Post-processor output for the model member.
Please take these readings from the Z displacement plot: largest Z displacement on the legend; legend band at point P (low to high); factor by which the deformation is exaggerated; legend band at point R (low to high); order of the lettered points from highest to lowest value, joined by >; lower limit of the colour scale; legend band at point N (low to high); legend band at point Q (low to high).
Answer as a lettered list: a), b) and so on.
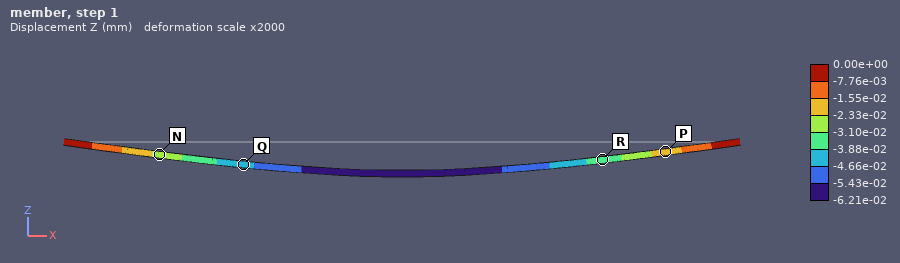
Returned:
a) 0.00e+00 mm
b) -2.33e-02 to -1.55e-02 mm
c) 2000
d) -3.88e-02 to -3.10e-02 mm
e) P > N > R > Q
f) -6.21e-02 mm
g) -3.10e-02 to -2.33e-02 mm
h) -4.66e-02 to -3.88e-02 mm
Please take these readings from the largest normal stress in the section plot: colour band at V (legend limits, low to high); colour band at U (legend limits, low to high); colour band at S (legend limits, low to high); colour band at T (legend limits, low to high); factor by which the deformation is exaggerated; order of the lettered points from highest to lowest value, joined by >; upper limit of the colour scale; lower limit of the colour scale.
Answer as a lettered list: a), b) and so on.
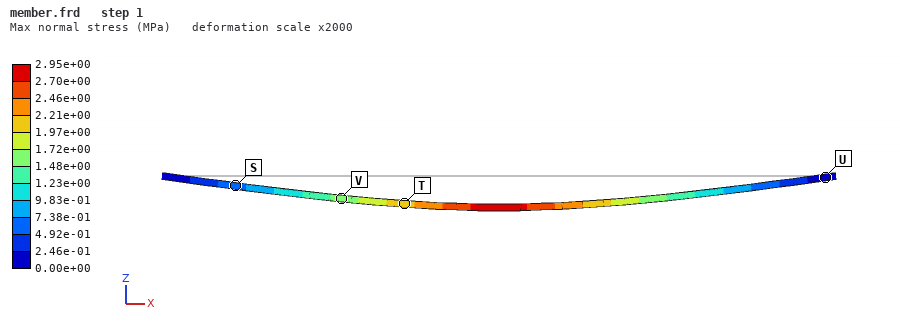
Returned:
a) 1.48e+00 to 1.72e+00 MPa
b) 0.00e+00 to 2.46e-01 MPa
c) 4.92e-01 to 7.38e-01 MPa
d) 1.97e+00 to 2.21e+00 MPa
e) 2000
f) T > V > S > U
g) 2.95e+00 MPa
h) 0.00e+00 MPa
